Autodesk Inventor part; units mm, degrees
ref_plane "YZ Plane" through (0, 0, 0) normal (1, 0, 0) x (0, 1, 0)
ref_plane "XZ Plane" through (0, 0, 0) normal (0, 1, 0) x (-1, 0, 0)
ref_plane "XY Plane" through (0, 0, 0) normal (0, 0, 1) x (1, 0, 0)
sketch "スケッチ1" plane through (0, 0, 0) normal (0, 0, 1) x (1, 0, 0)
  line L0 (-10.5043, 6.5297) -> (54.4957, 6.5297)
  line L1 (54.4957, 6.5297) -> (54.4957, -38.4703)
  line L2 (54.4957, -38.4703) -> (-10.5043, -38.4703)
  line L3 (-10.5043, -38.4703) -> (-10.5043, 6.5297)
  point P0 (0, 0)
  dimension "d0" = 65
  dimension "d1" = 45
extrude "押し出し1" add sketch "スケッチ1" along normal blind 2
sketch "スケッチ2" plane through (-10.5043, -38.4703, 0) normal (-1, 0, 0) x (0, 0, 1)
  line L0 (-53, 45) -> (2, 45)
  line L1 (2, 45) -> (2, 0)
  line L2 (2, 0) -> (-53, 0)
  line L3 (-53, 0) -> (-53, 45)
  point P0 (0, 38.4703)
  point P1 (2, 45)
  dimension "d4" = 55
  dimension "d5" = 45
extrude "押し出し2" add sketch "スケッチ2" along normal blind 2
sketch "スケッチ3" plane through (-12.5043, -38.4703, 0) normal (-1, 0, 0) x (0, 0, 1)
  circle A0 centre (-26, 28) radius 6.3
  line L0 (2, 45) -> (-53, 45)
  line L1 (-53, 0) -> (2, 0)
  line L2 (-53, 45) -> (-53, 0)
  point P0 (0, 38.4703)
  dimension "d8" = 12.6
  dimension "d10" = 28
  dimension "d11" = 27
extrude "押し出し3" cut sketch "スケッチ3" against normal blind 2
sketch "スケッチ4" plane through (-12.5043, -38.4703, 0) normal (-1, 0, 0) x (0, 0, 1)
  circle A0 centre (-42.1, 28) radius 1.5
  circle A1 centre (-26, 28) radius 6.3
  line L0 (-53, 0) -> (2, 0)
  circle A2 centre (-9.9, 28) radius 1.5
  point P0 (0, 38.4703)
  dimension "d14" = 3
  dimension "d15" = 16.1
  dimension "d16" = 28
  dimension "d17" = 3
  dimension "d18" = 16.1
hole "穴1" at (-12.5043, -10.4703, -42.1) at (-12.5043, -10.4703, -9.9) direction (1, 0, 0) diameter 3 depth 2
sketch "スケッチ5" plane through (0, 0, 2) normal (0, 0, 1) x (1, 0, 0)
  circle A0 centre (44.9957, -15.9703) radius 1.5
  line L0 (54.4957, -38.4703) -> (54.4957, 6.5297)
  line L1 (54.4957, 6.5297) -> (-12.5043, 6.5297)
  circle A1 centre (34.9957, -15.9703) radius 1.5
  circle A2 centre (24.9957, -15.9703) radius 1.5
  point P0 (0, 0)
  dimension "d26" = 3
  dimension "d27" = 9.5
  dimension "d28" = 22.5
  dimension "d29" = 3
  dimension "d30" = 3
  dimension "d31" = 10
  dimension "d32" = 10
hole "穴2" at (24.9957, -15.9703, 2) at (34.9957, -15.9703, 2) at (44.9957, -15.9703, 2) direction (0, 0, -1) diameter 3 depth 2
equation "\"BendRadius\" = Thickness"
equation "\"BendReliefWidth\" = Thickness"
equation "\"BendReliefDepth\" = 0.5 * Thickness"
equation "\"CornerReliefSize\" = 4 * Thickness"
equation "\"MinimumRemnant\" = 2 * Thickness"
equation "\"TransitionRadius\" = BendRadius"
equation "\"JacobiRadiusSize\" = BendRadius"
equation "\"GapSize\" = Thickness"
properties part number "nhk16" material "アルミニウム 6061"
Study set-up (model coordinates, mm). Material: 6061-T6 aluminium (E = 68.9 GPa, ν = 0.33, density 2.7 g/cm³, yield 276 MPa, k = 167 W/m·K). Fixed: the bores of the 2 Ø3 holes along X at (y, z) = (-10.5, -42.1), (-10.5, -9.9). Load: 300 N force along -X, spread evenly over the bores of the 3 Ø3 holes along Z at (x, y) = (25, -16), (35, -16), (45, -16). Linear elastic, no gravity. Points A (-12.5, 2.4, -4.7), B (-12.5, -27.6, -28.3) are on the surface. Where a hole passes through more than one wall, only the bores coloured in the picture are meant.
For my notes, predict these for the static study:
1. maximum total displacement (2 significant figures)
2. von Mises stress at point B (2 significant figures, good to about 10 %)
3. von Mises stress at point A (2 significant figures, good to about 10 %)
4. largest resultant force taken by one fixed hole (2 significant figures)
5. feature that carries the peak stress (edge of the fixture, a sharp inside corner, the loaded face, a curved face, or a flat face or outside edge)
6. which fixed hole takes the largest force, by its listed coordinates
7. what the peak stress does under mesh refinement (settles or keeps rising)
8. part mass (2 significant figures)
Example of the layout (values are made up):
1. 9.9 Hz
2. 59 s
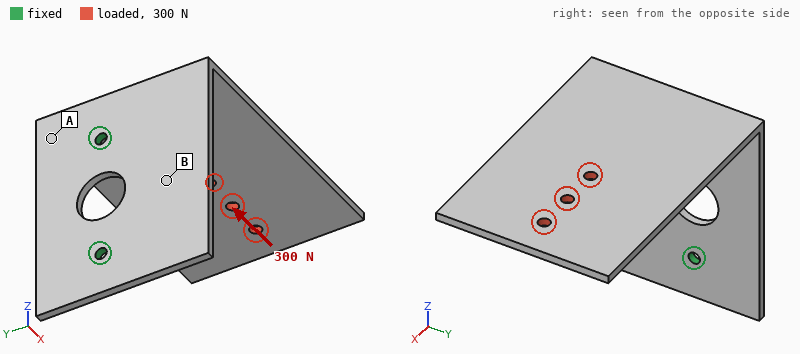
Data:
1. 1.0 mm
2. 20 MPa
3. 46 MPa
4. 330 N
5. edge of the fixture
6. (-10.5, -9.9)
7. keeps rising
8. 28 g
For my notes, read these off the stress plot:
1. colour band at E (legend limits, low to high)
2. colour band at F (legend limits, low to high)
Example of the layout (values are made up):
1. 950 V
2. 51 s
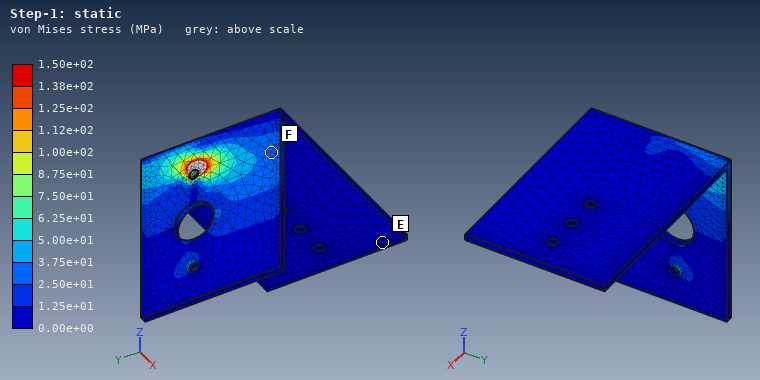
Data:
1. 0.00e+00 to 1.25e+01 MPa
2. 2.50e+01 to 3.75e+01 MPa
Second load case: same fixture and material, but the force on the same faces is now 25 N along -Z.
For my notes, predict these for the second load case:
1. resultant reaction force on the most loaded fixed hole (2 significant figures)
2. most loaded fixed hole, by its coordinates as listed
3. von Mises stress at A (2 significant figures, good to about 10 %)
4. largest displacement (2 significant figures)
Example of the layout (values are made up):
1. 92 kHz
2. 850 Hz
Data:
1. 27 N
2. (-10.5, -9.9)
3. 31 MPa
4. 1.1 mm
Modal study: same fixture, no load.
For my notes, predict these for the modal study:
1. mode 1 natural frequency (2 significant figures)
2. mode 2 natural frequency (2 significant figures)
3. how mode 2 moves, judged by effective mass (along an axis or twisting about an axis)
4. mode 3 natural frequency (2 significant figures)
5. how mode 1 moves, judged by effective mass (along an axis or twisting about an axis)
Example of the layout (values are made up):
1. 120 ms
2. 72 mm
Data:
1. 290 Hz
2. 480 Hz
3. along Y
4. 1200 Hz
5. along Z
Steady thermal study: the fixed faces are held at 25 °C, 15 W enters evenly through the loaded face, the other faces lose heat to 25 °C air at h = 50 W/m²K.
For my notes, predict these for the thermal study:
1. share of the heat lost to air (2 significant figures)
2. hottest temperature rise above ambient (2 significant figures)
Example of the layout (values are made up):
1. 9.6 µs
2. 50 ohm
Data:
1. 57 %
2. 40 K
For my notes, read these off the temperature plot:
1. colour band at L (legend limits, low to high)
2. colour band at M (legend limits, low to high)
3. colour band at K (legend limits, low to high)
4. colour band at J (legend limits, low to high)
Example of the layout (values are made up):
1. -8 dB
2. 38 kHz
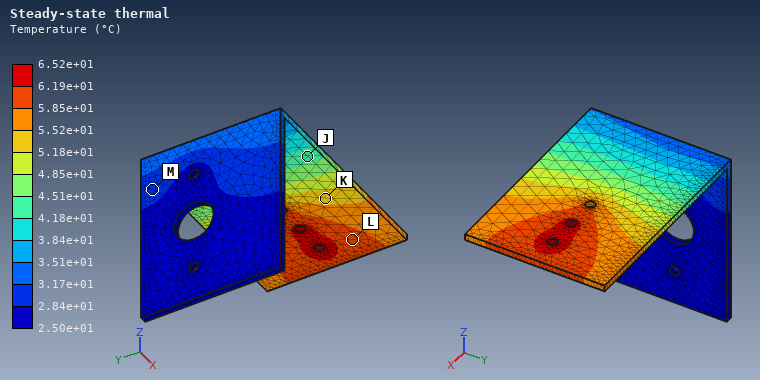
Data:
1. 5.85e+01 to 6.19e+01 °C
2. 2.84e+01 to 3.17e+01 °C
3. 5.18e+01 to 5.52e+01 °C
4. 4.18e+01 to 4.51e+01 °C
